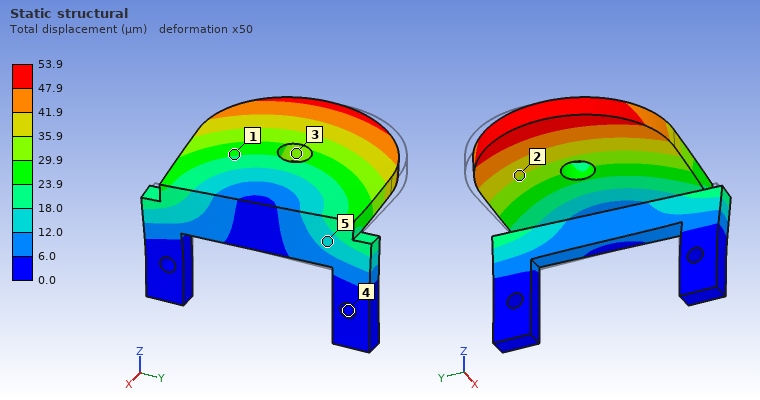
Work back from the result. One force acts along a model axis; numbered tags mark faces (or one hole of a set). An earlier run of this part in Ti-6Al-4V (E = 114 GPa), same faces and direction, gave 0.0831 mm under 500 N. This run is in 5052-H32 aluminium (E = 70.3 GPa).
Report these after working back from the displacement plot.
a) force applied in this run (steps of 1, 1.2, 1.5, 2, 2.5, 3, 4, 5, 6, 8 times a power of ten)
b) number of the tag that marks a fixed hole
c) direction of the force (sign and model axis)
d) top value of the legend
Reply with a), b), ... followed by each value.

a) 200 N
b) 4
c) -Y
d) 53.9 µm
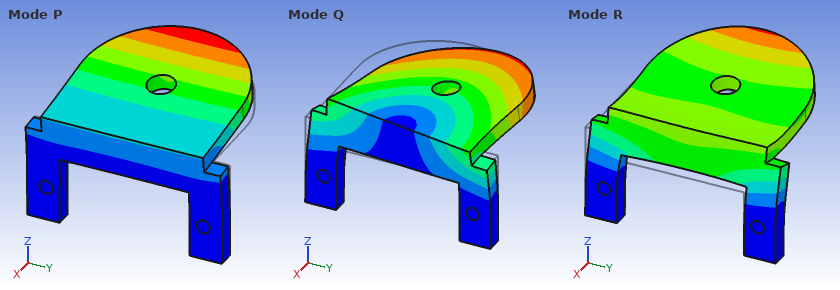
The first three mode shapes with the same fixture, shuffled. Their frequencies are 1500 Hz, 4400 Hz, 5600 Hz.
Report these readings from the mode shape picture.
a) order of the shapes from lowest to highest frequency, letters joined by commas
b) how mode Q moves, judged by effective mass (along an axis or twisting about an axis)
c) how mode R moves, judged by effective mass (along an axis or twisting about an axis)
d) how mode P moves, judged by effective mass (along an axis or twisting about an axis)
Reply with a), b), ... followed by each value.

a) P, Q, R
b) along Y
c) along X
d) along Z
